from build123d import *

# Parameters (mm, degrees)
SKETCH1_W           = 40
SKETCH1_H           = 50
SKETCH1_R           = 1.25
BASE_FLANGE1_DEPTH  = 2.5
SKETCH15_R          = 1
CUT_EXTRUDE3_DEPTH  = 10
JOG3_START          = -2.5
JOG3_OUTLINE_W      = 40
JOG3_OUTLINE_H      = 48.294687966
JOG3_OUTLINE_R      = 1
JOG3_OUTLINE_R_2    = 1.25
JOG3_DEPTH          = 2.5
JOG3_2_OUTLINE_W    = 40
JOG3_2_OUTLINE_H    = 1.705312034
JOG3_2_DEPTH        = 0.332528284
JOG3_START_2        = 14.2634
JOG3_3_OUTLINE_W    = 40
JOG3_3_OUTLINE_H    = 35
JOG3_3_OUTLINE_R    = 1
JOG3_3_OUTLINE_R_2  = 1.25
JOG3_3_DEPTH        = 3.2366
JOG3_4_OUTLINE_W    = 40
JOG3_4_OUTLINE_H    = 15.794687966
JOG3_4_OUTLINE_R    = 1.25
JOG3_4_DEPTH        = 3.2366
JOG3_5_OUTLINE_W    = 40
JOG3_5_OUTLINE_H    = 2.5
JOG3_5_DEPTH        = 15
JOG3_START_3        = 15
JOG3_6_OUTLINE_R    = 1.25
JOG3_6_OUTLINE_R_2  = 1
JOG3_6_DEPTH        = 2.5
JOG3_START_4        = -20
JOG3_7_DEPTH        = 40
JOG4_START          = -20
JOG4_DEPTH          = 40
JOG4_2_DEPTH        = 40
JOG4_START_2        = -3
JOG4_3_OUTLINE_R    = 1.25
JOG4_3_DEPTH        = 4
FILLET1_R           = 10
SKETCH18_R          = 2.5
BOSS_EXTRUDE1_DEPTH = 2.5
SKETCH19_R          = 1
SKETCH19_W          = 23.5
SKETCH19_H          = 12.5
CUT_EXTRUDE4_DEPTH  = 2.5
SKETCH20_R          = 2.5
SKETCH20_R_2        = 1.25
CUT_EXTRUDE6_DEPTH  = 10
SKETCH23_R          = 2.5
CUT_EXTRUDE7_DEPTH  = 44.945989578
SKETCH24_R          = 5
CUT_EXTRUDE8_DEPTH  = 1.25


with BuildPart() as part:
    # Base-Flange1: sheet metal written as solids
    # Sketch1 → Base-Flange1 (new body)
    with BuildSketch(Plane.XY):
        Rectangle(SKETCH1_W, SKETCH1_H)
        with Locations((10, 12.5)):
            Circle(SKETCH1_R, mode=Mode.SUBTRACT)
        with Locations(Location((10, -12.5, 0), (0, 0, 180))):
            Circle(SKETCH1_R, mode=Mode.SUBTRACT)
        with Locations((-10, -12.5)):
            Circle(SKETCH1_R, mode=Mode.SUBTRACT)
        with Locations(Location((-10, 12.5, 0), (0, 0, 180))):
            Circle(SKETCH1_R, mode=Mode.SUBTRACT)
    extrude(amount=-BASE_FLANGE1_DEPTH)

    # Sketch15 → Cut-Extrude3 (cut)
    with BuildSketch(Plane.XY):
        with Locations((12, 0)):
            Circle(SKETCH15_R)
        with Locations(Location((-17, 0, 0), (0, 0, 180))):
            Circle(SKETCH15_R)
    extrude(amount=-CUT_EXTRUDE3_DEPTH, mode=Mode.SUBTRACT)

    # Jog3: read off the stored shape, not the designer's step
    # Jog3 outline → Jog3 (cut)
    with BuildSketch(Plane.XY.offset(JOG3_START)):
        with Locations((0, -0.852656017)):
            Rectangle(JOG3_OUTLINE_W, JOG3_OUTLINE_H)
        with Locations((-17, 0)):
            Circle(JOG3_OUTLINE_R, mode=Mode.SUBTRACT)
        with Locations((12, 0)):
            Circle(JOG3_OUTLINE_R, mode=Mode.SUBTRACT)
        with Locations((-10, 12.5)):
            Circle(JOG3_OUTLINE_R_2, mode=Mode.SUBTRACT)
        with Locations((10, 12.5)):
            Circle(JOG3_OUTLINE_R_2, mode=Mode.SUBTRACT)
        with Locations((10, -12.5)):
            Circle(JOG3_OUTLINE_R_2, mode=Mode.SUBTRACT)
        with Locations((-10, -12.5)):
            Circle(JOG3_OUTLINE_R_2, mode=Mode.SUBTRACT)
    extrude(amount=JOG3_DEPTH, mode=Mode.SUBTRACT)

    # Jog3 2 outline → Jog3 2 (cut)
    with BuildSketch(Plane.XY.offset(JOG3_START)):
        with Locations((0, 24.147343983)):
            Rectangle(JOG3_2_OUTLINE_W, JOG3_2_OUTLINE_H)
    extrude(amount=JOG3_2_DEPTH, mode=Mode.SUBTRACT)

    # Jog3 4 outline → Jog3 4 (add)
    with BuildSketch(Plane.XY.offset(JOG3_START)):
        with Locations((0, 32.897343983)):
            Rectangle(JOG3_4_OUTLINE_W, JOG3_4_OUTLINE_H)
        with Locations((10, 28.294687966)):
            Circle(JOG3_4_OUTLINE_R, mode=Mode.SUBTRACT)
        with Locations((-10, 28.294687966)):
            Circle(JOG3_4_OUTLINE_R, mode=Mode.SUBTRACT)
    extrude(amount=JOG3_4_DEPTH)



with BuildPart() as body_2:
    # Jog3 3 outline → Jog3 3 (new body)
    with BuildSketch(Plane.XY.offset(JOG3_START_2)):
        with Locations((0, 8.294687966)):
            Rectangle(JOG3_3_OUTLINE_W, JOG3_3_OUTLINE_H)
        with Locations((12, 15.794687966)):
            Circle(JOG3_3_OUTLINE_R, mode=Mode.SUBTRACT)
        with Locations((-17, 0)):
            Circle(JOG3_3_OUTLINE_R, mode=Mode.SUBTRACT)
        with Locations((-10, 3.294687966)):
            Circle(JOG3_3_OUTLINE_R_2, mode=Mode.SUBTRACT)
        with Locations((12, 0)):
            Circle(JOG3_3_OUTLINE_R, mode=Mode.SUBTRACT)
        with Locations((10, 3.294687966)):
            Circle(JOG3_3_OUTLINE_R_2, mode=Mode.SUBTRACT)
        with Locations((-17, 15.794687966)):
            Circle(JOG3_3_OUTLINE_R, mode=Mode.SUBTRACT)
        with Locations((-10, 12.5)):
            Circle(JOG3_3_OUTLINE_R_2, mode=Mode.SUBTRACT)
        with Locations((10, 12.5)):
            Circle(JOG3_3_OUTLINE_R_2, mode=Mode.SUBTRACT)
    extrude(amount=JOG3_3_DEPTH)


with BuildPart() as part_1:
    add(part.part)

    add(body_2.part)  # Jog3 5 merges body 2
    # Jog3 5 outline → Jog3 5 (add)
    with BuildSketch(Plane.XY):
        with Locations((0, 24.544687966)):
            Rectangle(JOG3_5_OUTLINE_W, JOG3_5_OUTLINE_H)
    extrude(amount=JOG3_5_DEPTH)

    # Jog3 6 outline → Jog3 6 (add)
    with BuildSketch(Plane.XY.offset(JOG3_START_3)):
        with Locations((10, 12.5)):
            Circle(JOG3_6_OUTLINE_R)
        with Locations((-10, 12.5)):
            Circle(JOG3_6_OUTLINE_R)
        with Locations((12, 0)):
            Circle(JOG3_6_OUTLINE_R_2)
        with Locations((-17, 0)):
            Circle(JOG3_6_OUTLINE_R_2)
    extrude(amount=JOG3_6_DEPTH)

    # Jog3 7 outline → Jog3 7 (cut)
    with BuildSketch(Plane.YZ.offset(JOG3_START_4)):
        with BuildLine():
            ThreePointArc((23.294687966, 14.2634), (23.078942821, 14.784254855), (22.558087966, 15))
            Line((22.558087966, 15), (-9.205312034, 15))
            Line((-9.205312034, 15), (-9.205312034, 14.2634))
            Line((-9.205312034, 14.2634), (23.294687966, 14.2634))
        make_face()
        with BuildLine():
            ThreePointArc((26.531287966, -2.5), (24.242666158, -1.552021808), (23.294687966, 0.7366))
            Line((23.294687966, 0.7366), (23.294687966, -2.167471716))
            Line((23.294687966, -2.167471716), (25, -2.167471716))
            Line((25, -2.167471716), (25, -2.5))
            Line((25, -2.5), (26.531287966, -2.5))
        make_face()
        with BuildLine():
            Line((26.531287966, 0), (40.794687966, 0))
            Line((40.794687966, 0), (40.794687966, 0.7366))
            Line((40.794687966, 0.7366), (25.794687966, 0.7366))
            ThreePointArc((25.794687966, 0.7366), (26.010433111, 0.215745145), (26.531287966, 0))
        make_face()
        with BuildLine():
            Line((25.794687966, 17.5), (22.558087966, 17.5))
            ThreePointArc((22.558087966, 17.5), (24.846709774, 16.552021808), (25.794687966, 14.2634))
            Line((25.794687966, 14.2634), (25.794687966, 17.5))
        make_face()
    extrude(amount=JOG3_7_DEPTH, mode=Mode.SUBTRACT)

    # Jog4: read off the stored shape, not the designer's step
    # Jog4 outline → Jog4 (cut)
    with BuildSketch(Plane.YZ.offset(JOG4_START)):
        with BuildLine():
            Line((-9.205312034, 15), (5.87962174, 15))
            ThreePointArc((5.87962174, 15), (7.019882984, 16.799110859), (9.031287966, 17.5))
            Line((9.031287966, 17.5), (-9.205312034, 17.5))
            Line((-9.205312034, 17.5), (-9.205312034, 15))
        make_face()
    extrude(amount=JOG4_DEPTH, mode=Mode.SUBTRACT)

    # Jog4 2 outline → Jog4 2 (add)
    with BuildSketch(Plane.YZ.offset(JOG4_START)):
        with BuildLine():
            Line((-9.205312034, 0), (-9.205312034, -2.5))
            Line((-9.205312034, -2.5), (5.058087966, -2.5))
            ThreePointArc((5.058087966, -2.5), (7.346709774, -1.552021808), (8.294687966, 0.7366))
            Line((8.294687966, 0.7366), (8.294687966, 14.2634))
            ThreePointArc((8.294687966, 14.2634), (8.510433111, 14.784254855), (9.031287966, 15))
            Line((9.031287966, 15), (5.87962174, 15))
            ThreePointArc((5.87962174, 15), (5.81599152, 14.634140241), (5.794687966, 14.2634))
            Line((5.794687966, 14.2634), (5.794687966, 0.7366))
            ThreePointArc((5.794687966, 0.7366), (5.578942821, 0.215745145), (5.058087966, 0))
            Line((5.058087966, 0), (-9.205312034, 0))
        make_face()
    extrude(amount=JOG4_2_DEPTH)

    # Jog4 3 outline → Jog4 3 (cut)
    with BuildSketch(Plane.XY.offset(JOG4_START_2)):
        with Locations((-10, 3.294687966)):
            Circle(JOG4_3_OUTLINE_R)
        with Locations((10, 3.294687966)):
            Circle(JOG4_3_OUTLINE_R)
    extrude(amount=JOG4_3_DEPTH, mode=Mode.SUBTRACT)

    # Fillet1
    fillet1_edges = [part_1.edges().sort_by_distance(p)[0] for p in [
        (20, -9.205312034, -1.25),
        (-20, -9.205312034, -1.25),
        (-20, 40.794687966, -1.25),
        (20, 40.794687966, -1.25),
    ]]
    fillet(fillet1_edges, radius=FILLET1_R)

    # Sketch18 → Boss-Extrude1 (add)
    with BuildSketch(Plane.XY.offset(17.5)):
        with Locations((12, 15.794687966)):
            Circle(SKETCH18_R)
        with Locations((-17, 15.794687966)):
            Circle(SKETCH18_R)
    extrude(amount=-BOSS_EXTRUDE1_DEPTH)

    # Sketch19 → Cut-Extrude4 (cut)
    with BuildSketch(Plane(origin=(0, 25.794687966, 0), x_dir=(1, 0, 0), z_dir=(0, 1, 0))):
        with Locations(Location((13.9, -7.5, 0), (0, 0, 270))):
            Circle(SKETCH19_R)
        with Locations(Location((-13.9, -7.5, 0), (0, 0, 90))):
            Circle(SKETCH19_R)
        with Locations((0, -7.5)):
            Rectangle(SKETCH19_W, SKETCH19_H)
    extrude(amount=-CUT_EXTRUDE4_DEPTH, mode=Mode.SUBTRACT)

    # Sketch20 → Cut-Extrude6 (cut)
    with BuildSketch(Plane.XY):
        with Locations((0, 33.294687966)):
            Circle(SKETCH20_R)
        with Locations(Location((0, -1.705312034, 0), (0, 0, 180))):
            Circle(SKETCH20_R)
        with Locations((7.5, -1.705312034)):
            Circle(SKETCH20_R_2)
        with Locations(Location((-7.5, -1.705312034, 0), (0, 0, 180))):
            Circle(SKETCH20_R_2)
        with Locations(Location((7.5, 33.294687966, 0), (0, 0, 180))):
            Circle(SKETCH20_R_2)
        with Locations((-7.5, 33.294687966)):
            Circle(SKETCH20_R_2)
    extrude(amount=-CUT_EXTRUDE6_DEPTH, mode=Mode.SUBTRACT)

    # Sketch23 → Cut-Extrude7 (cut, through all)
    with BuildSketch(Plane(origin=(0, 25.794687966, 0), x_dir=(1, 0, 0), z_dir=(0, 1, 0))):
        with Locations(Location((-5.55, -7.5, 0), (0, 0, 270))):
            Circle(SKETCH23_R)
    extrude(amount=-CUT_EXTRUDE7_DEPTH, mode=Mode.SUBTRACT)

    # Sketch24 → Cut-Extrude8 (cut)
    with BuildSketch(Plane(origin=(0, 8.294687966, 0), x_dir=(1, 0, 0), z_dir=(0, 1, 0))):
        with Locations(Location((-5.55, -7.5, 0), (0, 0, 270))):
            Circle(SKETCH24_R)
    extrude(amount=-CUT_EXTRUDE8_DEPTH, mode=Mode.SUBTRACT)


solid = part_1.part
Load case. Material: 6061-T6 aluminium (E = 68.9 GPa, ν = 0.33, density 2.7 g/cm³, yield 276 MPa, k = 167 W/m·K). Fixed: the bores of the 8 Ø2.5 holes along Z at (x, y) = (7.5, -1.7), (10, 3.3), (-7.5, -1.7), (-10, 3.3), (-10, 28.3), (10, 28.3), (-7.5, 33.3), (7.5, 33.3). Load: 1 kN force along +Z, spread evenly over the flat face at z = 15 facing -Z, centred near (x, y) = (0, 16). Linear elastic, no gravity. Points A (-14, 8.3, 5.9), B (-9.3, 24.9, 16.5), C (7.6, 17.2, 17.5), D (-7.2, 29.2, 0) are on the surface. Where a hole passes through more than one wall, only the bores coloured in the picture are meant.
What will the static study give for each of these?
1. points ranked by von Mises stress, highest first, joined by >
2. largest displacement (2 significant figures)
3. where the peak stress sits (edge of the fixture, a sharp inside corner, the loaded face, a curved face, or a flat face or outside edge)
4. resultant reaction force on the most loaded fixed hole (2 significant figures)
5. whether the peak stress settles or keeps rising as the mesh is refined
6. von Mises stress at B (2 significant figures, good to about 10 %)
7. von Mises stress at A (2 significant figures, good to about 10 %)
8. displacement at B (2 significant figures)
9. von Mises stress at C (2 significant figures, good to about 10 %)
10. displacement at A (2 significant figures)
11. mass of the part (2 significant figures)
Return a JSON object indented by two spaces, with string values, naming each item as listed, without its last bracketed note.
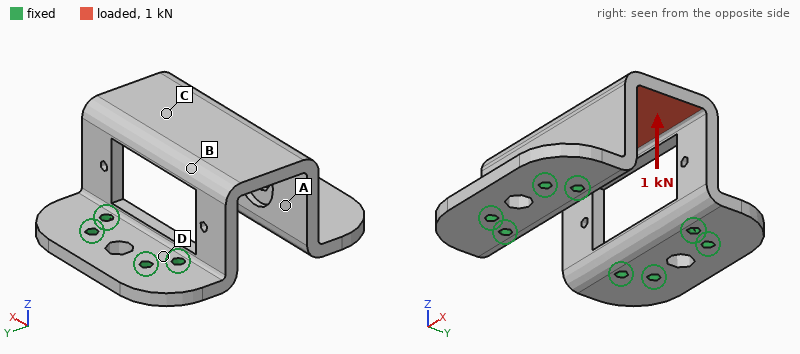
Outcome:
{
  "points ranked by von Mises stress, highest first, joined by >": "C > B > A > D",
  "largest displacement": "35 µm",
  "where the peak stress sits": "edge of the fixture",
  "resultant reaction force on the most loaded fixed hole": "280 N",
  "whether the peak stress settles or keeps rising as the mesh is refined": "keeps rising",
  "von Mises stress at B": "23 MPa",
  "von Mises stress at A": "13 MPa",
  "displacement at B": "23 µm",
  "von Mises stress at C": "36 MPa",
  "displacement at A": "5.5 µm",
  "mass of the part": "19 g"
}
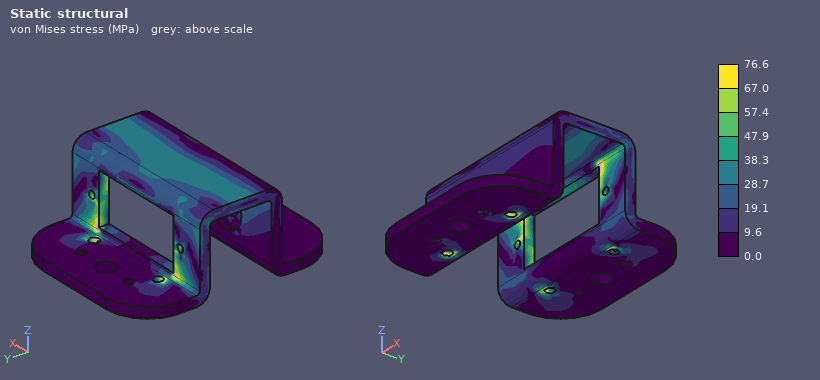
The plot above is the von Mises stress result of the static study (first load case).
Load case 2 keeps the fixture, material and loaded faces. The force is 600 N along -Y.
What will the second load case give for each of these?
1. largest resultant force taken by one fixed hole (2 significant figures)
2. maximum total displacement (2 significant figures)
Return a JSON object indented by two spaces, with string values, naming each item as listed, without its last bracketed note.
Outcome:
{
  "largest resultant force taken by one fixed hole": "160 N",
  "maximum total displacement": "92 µm"
}
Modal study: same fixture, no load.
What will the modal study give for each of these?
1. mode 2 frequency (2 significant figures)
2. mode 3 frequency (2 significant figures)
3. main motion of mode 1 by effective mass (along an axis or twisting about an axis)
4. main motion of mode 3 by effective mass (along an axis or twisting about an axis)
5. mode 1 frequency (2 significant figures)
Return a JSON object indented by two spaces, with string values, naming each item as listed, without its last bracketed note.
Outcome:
{
  "mode 2 frequency": "6000 Hz",
  "mode 3 frequency": "10 kHz",
  "main motion of mode 1 by effective mass": "along Y",
  "main motion of mode 3 by effective mass": "along X",
  "mode 1 frequency": "4900 Hz"
}
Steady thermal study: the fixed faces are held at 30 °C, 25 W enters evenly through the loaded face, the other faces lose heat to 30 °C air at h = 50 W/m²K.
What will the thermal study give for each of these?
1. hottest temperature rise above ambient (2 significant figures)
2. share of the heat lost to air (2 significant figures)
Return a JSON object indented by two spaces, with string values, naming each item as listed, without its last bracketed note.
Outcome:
{
  "hottest temperature rise above ambient": "29 K",
  "share of the heat lost to air": "12 %"
}
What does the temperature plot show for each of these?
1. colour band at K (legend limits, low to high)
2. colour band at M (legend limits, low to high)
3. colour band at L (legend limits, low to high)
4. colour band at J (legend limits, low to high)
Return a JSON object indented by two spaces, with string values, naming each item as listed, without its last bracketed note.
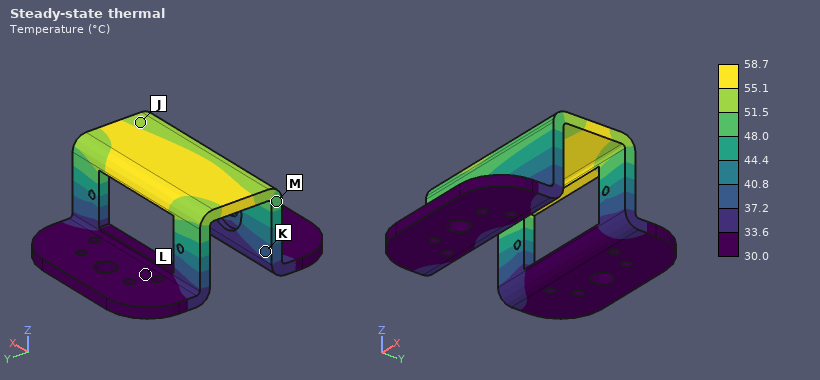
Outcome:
{
  "colour band at K": "37.2 to 40.8 °C",
  "colour band at M": "48.0 to 51.5 °C",
  "colour band at L": "30.0 to 33.6 °C",
  "colour band at J": "51.5 to 55.1 °C"
}
